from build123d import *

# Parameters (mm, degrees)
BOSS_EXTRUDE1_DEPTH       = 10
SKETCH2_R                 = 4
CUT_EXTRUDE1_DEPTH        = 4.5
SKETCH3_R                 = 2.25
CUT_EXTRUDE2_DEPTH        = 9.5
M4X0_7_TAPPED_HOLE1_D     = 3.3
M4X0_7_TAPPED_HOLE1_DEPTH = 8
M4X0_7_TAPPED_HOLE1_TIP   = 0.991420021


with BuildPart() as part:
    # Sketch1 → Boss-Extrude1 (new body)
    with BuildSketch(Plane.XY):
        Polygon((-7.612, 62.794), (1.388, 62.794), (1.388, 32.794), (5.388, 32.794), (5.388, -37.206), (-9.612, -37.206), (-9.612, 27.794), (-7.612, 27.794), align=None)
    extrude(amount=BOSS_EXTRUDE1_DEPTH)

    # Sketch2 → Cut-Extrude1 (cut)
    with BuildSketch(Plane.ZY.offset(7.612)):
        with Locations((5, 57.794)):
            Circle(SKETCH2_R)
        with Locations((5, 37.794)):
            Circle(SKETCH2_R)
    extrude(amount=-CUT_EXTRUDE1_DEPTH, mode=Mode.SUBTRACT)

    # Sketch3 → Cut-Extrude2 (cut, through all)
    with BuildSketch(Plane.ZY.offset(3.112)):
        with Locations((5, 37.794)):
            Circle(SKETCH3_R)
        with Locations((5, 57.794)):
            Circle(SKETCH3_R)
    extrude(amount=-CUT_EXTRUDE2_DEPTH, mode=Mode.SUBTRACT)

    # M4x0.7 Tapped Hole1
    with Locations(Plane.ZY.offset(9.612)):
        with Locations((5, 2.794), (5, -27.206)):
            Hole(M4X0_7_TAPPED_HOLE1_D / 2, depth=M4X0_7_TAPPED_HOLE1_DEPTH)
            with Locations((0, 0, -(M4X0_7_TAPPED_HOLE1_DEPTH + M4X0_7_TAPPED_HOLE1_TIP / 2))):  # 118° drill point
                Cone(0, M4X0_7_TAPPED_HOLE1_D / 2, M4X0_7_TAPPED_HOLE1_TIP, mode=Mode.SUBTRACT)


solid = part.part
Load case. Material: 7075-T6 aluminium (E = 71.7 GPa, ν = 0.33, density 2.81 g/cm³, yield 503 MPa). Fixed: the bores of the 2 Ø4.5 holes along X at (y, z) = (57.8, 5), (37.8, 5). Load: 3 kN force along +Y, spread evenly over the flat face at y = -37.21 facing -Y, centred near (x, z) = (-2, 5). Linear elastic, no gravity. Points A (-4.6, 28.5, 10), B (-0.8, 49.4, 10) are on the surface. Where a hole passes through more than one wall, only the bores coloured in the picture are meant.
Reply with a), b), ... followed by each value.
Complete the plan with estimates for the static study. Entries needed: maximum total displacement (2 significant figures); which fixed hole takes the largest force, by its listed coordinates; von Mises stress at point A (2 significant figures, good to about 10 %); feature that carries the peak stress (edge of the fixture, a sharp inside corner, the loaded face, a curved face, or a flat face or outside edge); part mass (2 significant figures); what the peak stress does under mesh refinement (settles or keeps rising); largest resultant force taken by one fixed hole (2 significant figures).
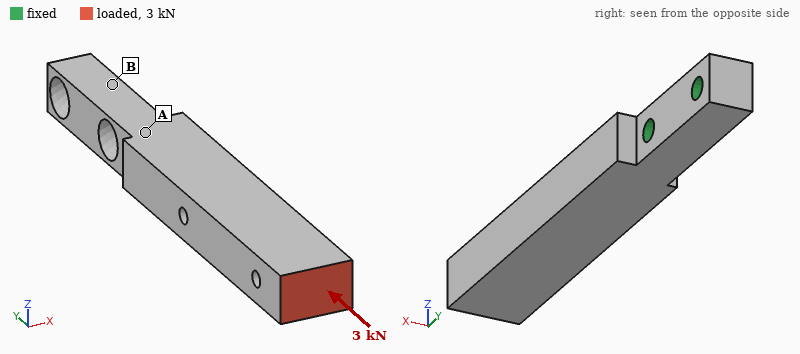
a) 67 µm
b) (37.8, 5)
c) 30 MPa
d) edge of the fixture
e) 35 g
f) keeps rising
g) 2.7 kN
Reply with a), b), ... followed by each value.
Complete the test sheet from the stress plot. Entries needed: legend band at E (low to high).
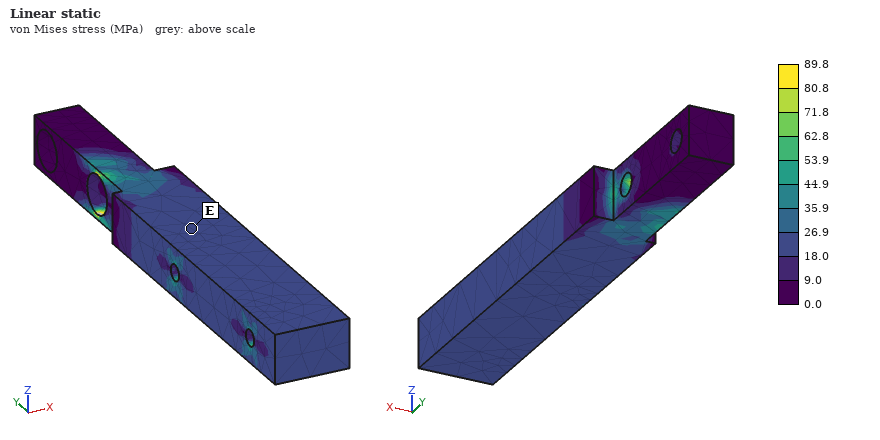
a) 18.0 to 26.9 MPa
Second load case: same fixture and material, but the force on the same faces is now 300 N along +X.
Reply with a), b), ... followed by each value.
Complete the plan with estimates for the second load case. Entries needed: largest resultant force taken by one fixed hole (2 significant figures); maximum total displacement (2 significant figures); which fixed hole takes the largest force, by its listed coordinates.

a) 1.1 kN
b) 0.76 mm
c) (37.8, 5)
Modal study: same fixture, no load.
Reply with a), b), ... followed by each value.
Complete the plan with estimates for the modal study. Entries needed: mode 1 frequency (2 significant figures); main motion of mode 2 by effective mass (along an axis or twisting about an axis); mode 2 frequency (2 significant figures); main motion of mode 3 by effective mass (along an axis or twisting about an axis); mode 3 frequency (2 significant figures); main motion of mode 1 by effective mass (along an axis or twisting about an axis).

a) 1000 Hz
b) along Z
c) 1100 Hz
d) twisting about Y
e) 6800 Hz
f) along X
